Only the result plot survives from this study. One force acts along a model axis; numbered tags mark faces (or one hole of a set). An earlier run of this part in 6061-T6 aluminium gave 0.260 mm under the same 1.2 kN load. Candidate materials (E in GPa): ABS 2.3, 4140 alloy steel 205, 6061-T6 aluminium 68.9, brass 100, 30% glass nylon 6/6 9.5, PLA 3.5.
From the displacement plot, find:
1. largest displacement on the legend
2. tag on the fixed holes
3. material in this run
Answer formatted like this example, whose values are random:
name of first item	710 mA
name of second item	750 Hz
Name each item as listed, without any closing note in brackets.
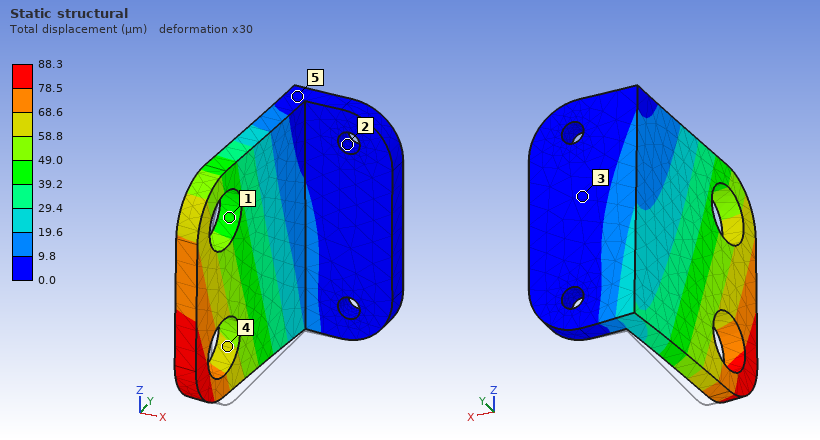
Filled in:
largest displacement on the legend	88.3 µm
tag on the fixed holes	2
material in this run	4140 alloy steel
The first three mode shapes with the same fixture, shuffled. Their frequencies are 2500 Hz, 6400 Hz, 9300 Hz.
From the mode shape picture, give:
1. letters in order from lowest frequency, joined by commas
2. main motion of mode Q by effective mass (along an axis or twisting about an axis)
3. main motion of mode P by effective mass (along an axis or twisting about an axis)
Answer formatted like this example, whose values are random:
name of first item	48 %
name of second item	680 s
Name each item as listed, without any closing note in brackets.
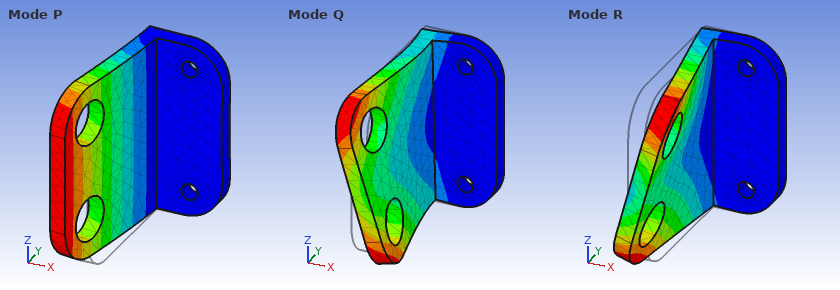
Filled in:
letters in order from lowest frequency, joined by commas	P, R, Q
main motion of mode Q by effective mass	along Z
main motion of mode P by effective mass	along X
